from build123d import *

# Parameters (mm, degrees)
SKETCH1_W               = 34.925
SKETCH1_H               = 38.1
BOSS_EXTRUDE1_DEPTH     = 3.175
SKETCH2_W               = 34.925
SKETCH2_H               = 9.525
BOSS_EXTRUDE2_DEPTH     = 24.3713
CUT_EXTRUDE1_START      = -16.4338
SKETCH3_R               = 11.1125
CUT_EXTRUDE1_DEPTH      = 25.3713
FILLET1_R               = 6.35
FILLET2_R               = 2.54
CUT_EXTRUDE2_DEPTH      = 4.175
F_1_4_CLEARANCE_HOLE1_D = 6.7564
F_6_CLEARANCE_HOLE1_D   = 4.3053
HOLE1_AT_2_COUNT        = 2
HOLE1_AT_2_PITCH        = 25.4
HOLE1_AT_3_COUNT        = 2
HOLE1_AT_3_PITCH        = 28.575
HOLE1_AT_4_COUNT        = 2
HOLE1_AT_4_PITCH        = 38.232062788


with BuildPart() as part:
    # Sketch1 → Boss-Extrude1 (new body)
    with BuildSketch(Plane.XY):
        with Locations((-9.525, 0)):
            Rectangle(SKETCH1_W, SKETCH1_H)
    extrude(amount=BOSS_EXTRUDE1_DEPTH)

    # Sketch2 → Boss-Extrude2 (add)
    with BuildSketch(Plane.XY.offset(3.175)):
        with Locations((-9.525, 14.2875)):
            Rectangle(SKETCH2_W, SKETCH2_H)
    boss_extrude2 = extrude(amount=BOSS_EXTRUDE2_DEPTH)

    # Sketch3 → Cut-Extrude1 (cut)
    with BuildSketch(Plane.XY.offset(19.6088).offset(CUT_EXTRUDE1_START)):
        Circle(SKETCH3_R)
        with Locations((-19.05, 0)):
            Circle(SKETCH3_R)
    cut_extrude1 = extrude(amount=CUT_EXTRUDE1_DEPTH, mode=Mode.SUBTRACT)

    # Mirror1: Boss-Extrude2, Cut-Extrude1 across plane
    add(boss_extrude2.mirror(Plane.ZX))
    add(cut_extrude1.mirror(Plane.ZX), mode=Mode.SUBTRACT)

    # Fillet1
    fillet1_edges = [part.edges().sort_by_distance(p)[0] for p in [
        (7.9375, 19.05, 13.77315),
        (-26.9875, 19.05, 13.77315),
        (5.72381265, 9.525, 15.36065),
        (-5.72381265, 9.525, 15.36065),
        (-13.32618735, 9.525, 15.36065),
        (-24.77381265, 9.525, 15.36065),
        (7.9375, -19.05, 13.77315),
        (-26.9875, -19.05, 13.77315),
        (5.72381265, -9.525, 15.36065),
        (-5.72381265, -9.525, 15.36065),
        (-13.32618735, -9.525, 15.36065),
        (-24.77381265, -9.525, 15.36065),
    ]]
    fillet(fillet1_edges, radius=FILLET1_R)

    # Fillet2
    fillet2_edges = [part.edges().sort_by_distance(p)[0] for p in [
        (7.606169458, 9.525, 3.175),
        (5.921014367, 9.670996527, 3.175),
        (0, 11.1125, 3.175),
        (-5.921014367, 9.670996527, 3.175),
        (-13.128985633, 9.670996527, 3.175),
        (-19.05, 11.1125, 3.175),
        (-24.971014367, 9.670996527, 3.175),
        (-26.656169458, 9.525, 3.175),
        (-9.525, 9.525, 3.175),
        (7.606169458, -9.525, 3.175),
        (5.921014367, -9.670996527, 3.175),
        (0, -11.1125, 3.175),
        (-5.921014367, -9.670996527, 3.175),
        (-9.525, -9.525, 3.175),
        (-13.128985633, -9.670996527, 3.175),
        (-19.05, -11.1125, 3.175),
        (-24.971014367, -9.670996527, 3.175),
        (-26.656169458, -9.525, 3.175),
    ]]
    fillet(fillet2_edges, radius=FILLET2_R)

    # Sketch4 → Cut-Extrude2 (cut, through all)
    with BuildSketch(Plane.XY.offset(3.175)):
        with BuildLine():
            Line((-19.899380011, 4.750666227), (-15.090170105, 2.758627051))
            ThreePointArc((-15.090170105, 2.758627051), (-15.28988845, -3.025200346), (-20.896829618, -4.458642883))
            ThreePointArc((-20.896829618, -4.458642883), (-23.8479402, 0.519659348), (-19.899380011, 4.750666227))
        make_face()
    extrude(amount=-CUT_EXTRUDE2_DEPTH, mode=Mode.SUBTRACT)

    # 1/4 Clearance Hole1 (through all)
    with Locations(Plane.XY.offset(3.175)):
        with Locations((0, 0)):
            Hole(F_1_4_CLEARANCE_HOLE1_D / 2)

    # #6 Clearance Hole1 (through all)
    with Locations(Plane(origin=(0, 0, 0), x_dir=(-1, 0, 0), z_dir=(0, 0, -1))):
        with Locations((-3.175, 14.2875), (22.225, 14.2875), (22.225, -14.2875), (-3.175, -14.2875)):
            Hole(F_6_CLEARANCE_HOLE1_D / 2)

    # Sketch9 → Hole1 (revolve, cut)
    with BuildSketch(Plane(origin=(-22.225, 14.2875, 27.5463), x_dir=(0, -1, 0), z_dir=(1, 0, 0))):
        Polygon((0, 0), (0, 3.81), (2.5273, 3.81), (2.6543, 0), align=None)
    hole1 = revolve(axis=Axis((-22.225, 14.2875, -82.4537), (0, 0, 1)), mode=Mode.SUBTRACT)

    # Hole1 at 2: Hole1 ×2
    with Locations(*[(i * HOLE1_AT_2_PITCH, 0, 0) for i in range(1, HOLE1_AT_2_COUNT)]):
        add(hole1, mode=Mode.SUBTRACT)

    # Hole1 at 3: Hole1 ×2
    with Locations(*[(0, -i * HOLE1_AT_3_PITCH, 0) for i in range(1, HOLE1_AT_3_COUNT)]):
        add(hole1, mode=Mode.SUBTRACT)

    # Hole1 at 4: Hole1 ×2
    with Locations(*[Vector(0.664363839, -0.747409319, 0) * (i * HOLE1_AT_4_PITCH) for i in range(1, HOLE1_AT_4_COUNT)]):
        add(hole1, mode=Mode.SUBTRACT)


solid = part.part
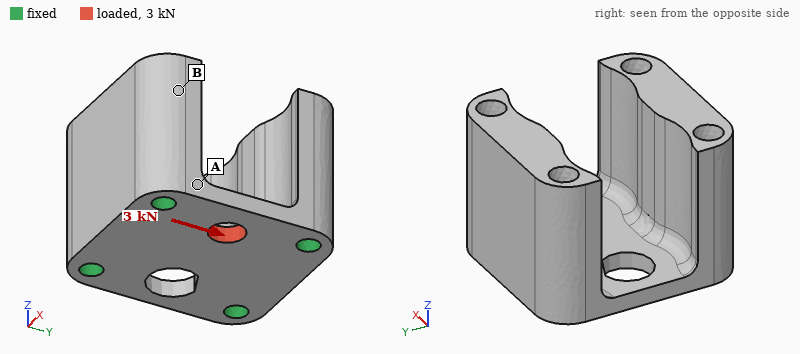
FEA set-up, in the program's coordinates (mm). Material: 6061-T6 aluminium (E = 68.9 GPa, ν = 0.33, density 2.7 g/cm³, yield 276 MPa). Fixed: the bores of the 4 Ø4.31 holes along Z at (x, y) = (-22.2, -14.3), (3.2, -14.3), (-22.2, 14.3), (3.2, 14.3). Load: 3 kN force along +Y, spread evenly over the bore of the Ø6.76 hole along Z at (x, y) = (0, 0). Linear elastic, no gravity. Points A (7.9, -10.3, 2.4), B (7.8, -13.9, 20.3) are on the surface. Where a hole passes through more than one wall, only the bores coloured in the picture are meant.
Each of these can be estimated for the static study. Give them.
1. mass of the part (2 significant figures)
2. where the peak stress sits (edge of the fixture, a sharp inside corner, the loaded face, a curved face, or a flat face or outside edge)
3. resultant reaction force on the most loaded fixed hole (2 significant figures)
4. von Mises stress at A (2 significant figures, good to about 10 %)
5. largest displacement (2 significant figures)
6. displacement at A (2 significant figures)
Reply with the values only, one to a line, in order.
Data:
44 g
the loaded face
1.2 kN
17 MPa
6.8 µm
1.7 µm
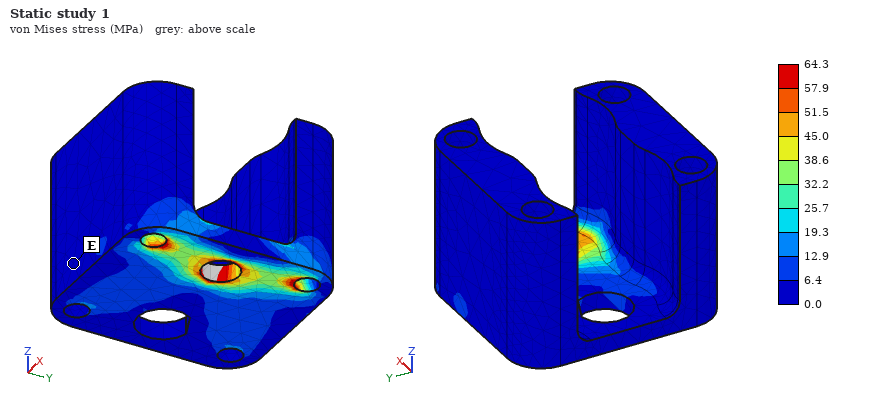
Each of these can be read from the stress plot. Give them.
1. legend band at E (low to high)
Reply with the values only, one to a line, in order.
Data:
0.0 to 6.4 MPa
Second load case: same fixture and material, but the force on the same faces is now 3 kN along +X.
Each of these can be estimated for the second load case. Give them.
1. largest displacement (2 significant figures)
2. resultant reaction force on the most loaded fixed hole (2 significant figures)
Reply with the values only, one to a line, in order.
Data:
16 µm
920 N
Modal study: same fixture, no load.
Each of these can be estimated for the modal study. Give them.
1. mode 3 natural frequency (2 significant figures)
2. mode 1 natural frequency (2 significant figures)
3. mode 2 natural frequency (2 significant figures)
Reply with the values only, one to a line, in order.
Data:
40 kHz
34 kHz
38 kHz
